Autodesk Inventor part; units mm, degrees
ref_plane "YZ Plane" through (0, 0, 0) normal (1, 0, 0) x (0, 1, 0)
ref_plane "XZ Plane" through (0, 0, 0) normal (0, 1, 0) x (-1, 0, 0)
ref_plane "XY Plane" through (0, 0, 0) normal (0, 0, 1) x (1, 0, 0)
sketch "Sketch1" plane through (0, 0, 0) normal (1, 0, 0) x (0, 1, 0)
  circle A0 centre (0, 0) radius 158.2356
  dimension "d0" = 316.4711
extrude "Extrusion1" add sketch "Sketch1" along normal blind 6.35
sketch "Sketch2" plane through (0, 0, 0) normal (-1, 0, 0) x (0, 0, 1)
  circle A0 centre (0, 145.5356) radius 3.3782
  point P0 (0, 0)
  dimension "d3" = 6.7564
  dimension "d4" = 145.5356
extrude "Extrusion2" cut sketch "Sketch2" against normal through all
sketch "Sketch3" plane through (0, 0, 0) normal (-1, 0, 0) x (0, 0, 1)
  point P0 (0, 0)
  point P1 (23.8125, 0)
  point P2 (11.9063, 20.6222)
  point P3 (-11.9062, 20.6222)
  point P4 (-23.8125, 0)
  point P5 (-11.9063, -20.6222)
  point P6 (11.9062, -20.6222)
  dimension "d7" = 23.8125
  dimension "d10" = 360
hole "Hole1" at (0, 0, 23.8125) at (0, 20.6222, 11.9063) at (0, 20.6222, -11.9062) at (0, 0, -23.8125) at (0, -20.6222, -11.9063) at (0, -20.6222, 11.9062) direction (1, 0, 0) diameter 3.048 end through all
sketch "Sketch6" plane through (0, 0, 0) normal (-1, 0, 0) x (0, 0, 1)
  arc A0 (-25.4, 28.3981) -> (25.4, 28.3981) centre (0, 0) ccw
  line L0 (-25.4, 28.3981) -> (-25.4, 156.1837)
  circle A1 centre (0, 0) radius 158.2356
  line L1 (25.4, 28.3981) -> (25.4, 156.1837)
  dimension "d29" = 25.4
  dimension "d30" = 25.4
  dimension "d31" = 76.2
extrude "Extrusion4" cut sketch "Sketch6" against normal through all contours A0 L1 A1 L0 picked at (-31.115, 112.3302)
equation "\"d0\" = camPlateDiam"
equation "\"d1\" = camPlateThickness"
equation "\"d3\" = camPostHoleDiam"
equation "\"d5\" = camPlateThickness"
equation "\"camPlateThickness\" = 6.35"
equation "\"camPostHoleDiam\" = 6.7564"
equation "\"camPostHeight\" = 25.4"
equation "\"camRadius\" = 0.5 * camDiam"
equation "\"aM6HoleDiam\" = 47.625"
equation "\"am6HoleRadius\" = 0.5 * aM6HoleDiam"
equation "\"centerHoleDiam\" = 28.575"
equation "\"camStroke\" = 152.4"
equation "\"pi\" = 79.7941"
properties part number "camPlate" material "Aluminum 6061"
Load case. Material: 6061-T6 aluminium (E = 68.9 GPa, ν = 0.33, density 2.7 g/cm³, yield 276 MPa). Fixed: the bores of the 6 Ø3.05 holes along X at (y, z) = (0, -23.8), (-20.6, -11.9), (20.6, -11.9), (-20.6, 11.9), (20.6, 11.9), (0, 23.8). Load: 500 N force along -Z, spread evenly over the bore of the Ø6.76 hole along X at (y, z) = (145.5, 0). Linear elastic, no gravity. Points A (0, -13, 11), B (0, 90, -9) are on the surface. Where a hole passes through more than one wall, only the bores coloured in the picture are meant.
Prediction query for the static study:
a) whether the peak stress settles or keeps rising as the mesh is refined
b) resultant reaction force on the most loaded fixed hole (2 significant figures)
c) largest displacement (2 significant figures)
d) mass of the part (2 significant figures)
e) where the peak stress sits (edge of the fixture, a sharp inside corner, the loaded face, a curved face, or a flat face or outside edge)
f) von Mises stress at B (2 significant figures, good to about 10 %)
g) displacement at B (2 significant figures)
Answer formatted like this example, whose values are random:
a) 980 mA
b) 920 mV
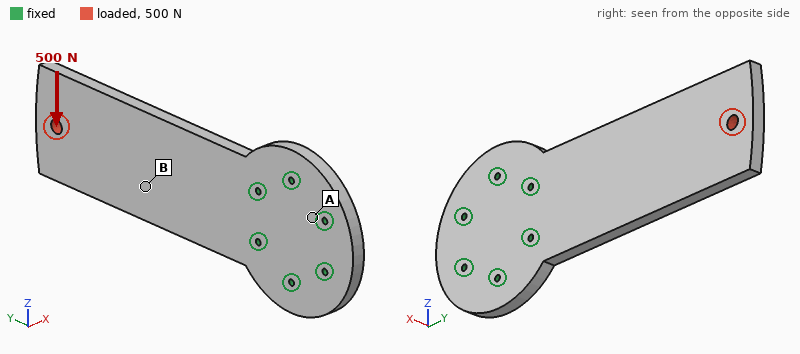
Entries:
a) keeps rising
b) 1.1 kN
c) 96 µm
d) 180 g
e) edge of the fixture
f) 5.1 MPa
g) 35 µm
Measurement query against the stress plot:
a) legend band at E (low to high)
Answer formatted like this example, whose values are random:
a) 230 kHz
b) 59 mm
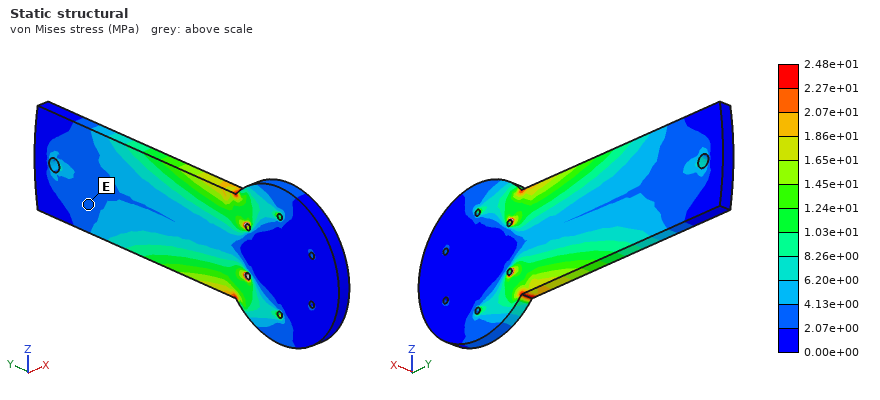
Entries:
a) 2.07e+00 to 4.13e+00 MPa
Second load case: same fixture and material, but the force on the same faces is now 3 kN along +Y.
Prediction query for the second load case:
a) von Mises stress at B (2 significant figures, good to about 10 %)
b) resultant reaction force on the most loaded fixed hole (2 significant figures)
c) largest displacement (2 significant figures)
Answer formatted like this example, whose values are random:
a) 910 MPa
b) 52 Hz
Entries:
a) 9.4 MPa
b) 1.1 kN
c) 22 µm
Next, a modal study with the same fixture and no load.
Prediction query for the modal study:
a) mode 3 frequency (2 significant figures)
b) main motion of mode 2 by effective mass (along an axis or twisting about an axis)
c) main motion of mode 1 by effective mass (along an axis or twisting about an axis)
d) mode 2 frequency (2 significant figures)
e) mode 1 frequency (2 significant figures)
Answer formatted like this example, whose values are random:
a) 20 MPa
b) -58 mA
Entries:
a) 1700 Hz
b) twisting about Y
c) along X
d) 1500 Hz
e) 280 Hz
